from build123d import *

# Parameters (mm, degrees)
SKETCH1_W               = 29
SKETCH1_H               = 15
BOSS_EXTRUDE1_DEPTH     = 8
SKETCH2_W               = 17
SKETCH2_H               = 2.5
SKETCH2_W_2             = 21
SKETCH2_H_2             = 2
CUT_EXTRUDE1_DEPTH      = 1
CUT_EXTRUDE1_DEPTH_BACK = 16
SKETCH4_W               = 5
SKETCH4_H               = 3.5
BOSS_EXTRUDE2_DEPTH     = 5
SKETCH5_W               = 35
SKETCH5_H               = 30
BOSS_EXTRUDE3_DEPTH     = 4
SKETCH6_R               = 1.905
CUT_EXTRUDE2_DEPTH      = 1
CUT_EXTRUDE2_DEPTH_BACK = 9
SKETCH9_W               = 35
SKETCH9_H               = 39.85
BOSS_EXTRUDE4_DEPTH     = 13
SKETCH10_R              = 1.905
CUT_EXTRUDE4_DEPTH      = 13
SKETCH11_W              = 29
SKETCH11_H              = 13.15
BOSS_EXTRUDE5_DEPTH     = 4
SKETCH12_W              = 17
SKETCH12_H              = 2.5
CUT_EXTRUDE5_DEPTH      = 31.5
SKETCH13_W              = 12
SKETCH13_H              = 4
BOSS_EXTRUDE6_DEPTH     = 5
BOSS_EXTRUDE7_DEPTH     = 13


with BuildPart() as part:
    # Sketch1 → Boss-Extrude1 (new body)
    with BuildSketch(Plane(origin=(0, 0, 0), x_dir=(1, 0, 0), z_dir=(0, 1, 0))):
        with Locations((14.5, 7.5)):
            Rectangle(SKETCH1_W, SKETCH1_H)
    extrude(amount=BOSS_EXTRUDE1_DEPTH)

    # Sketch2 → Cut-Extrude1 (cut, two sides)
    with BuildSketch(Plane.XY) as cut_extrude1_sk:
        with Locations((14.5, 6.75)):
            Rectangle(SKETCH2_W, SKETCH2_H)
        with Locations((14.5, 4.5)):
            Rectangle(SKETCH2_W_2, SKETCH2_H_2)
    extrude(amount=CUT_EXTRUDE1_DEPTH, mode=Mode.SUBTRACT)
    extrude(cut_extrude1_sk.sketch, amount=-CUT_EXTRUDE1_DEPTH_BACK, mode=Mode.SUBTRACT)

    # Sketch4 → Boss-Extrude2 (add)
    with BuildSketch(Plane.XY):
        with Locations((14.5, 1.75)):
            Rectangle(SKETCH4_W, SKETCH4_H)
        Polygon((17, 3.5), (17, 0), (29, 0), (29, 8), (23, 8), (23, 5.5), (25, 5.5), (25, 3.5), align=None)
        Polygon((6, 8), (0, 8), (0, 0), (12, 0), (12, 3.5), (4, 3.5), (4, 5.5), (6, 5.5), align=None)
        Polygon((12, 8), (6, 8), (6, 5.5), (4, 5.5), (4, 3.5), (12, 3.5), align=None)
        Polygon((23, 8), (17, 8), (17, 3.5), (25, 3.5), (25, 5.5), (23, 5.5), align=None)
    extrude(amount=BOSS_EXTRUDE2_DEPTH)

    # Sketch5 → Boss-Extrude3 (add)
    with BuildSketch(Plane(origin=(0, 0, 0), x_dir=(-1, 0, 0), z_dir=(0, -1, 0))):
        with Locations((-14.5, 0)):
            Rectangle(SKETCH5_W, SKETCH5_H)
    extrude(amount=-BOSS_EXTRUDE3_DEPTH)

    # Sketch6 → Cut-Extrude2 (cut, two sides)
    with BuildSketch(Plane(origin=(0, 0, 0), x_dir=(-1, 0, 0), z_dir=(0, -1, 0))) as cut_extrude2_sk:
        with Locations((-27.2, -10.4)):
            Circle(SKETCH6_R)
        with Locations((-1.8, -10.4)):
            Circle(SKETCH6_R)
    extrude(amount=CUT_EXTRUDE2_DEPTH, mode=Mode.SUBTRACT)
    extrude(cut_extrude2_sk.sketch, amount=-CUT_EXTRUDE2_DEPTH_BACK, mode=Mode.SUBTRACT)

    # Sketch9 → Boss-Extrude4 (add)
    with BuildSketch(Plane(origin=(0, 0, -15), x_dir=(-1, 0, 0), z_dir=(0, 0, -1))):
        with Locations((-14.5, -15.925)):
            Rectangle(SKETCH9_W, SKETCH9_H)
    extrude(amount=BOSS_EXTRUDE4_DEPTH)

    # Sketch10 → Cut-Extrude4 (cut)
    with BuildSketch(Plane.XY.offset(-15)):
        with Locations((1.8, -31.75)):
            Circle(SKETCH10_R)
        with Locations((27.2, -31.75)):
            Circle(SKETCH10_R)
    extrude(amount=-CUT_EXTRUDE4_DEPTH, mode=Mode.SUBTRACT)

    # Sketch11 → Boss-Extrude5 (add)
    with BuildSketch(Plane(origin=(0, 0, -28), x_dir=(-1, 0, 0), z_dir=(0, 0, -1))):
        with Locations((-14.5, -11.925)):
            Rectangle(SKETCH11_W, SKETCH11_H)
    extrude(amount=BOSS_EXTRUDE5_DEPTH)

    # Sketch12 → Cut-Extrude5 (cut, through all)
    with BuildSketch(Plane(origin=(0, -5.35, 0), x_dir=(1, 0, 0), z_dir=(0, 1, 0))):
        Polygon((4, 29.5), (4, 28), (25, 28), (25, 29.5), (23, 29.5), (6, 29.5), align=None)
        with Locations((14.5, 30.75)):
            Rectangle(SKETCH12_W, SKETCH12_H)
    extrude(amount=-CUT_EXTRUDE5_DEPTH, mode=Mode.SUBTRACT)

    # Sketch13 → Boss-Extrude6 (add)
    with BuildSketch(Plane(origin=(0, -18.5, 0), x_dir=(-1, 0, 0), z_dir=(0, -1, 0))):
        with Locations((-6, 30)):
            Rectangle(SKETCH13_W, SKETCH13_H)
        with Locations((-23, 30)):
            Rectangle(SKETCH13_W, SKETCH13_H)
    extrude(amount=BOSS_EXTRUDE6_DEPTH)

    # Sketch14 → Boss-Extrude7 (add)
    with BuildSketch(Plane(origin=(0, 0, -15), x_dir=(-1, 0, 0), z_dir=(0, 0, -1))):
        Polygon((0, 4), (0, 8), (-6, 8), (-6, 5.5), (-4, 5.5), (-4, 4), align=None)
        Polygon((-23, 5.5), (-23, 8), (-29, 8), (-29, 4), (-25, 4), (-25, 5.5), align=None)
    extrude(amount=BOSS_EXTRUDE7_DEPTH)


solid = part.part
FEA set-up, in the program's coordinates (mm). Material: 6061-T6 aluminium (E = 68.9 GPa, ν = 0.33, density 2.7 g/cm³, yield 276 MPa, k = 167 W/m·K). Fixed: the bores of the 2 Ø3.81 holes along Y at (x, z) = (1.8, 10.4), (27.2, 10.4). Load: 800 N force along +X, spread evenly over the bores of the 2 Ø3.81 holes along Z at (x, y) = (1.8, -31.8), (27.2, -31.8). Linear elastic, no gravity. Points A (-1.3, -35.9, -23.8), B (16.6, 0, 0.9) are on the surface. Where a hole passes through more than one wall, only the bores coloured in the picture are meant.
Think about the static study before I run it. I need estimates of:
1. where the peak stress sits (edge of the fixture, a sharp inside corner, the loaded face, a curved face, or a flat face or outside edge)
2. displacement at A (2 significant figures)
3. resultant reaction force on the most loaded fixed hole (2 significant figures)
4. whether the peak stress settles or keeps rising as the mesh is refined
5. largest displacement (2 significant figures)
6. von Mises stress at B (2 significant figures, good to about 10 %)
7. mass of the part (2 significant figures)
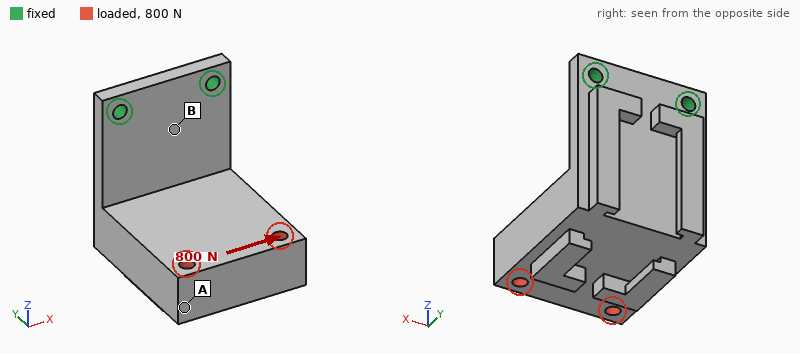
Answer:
edge of the fixture
0.45 mm
1.4 kN
keeps rising
0.46 mm
120 MPa
67 g
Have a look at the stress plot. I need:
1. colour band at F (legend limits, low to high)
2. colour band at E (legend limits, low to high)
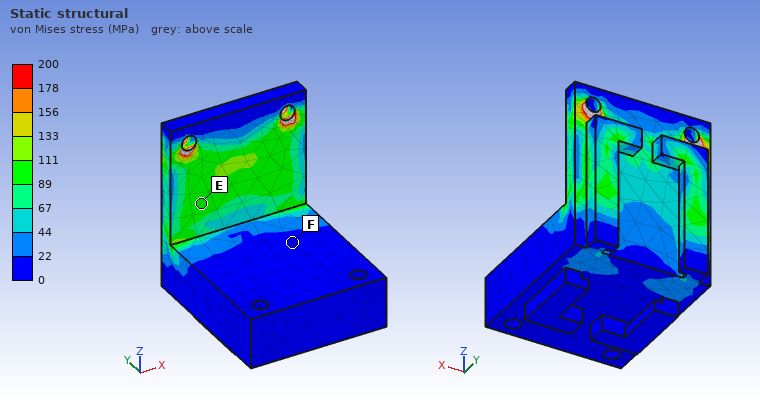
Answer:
0 to 22 MPa
89 to 111 MPa
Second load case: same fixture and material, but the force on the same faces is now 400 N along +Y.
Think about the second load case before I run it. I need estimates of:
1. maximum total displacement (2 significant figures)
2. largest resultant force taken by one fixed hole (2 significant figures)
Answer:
0.46 mm
200 N
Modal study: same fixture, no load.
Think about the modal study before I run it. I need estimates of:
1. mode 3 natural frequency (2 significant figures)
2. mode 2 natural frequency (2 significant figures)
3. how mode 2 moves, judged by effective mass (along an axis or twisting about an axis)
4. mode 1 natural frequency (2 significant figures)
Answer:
3200 Hz
1500 Hz
along X
670 Hz
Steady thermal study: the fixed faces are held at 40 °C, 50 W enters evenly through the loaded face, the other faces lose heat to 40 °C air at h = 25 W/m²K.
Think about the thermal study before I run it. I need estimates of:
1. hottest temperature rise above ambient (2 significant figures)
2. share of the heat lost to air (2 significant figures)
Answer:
68 K
18 %
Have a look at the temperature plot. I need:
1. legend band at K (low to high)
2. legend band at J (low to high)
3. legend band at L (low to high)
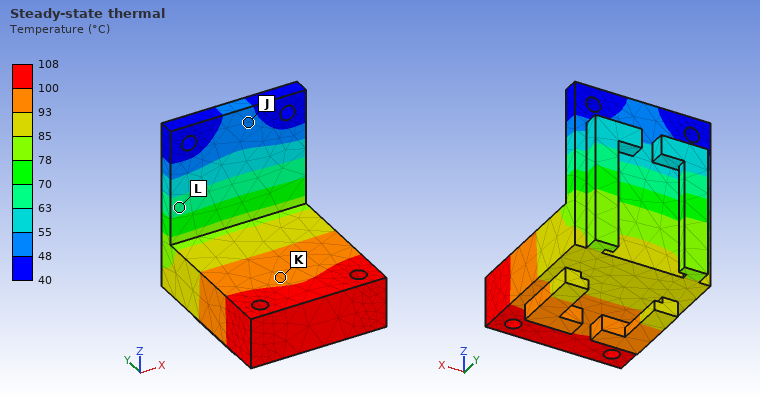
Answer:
93 to 100 °C
48 to 55 °C
63 to 70 °C
